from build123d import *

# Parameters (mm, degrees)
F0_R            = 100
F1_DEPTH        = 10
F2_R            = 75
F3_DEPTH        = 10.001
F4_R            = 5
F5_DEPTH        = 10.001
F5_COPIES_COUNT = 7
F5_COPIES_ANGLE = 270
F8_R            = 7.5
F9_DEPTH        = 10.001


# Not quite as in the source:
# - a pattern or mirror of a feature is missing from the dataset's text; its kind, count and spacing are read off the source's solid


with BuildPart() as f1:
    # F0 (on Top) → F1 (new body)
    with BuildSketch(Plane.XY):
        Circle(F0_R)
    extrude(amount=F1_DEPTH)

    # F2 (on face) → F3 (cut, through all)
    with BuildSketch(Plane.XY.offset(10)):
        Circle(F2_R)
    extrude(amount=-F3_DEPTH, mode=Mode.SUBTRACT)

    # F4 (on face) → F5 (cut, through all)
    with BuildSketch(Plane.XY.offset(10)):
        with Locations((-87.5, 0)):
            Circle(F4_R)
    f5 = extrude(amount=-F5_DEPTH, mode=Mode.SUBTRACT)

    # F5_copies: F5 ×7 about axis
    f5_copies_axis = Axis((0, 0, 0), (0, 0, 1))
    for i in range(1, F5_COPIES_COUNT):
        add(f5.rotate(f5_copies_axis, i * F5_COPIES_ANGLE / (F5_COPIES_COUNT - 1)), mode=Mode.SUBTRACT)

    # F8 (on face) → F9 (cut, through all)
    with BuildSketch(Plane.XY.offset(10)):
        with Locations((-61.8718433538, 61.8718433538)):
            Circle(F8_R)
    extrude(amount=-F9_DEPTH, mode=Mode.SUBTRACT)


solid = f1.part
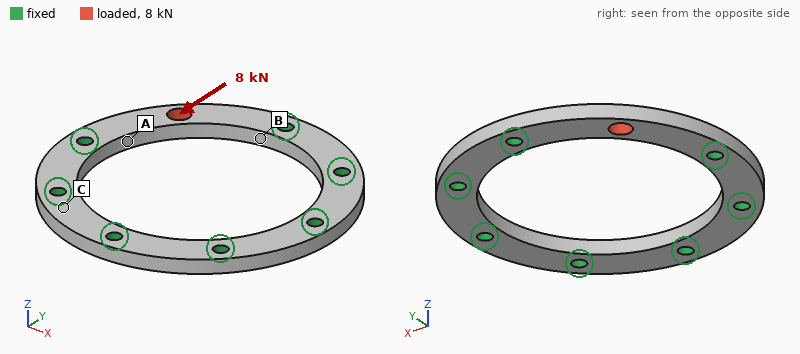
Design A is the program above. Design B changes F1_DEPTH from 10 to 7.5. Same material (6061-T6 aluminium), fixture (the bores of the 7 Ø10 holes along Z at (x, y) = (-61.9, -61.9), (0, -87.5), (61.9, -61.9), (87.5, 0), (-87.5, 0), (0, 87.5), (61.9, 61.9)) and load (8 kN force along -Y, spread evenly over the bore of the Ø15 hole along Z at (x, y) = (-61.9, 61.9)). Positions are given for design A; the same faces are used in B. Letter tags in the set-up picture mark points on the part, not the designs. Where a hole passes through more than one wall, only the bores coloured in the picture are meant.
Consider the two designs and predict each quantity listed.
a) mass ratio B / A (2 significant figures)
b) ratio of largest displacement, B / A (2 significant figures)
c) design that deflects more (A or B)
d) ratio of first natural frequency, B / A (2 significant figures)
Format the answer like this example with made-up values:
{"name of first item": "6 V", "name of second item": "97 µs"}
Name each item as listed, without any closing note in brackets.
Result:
{"mass ratio B / A": "0.75", "ratio of largest displacement, B / A": "1.3", "design that deflects more": "B", "ratio of first natural frequency, B / A": "0.77"}
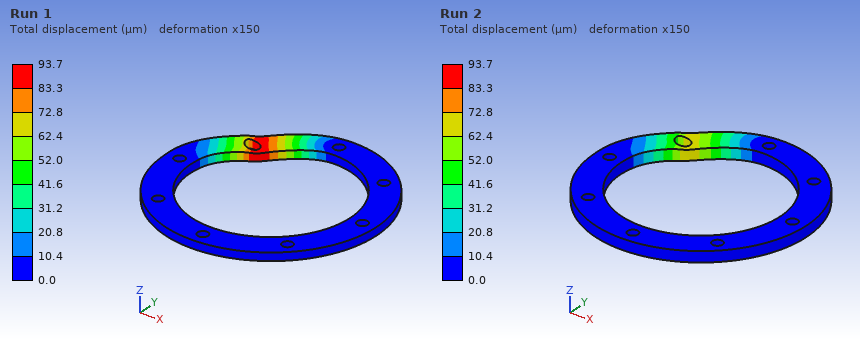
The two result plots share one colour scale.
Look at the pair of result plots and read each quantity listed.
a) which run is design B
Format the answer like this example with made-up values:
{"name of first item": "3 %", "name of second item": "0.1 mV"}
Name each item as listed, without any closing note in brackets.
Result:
{"which run is design B": "Run 1"}
